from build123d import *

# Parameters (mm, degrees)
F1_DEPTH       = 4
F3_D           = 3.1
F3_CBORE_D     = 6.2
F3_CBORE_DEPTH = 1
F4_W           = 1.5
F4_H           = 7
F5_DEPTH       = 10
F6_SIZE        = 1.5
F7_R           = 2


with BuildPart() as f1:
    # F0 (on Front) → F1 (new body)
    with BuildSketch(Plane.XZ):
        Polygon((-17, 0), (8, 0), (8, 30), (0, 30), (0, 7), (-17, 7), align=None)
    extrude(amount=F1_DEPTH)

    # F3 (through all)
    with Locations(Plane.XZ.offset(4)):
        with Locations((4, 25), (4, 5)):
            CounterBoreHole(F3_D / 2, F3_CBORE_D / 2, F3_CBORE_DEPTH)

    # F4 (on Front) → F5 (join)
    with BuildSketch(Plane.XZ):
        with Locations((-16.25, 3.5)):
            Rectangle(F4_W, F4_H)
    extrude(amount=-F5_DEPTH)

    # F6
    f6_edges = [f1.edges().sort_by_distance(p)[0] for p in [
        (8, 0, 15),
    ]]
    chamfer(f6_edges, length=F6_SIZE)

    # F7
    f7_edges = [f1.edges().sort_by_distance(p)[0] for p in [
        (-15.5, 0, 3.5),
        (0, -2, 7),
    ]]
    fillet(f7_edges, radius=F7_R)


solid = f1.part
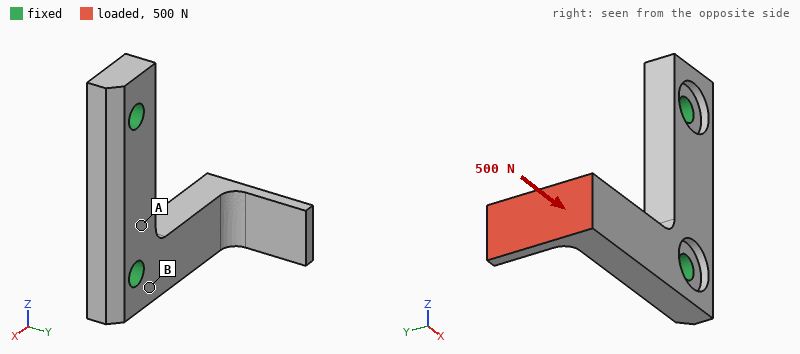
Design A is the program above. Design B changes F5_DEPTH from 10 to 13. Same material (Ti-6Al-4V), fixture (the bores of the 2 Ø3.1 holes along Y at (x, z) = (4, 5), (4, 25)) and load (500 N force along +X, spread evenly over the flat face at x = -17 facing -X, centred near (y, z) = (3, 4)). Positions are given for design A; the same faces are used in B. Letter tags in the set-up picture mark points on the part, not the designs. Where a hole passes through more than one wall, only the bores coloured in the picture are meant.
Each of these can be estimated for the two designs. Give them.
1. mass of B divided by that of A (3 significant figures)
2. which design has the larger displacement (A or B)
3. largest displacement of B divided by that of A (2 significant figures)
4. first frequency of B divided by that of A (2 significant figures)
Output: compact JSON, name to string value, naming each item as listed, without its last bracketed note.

{"mass of B divided by that of A": "1.02", "which design has the larger displacement": "B", "largest displacement of B divided by that of A": "1.9", "first frequency of B divided by that of A": "0.88"}
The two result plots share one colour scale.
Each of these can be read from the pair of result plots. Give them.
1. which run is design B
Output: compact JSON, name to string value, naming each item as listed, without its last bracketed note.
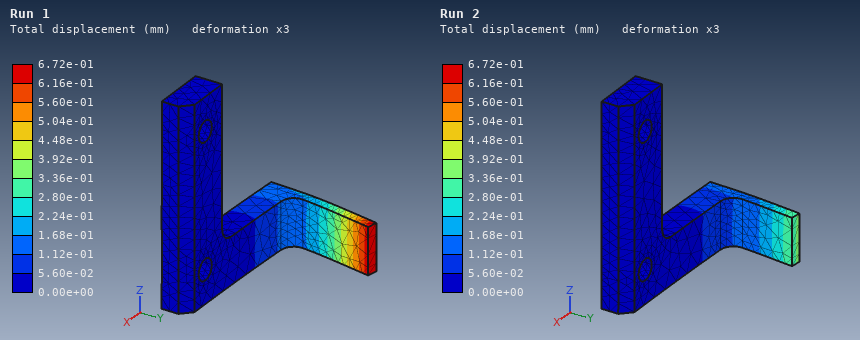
{"which run is design B": "Run 1"}
